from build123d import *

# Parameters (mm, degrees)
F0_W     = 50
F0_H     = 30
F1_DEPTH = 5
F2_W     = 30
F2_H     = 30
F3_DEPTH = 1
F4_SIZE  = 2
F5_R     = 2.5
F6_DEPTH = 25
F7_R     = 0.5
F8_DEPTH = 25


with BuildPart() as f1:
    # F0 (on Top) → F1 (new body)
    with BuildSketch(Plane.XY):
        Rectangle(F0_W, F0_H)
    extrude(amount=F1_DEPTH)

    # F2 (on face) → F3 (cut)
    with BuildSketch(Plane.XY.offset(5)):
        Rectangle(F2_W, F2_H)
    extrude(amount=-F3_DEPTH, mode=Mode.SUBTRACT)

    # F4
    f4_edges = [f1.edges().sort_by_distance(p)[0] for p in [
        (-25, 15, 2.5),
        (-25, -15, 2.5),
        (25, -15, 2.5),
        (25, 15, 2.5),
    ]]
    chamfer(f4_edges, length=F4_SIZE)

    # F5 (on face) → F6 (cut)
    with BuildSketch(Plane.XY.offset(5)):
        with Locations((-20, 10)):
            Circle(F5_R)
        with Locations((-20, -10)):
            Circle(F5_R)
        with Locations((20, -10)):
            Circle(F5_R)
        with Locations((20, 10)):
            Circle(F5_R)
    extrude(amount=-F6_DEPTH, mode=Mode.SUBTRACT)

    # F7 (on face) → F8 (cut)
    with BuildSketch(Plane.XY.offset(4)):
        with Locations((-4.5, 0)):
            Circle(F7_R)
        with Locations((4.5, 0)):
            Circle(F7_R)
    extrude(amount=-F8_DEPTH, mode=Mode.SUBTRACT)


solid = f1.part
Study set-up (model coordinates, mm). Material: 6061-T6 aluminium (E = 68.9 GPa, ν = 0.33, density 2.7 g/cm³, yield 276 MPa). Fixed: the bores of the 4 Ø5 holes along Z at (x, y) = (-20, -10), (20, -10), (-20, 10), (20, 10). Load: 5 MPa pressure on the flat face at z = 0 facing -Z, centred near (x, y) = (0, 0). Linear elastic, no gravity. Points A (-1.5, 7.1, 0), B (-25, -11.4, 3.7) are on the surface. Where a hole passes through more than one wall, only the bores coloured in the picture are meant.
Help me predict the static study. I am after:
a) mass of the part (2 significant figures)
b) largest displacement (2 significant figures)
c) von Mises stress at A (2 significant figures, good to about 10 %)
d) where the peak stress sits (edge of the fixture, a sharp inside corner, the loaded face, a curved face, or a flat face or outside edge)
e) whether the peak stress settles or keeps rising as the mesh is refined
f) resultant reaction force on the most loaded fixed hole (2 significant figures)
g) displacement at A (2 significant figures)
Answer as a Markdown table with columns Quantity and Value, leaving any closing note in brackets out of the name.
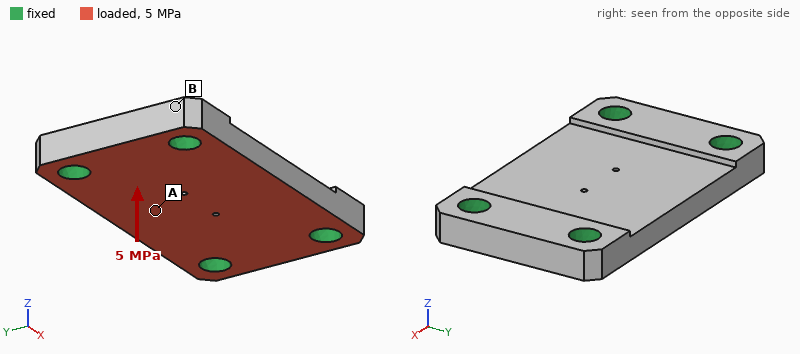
| Quantity | Value |
|---|---|
| mass of the part | 17 g |
| largest displacement | 68 µm |
| von Mises stress at A | 90 MPa |
| where the peak stress sits | edge of the fixture |
| whether the peak stress settles or keeps rising as the mesh is refined | keeps rising |
| resultant reaction force on the most loaded fixed hole | 1.8 kN |
| displacement at A | 64 µm |
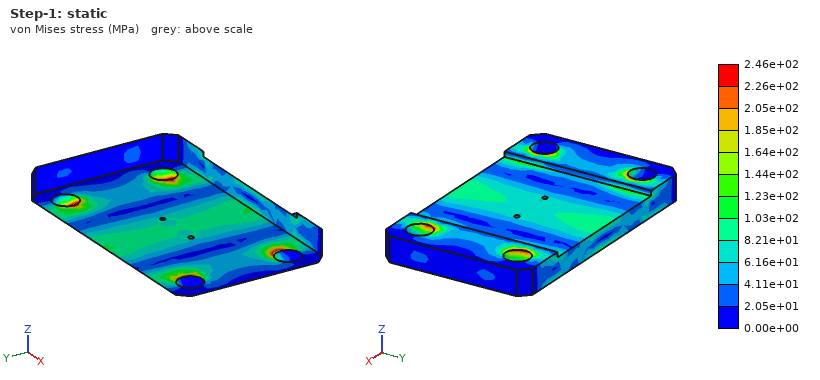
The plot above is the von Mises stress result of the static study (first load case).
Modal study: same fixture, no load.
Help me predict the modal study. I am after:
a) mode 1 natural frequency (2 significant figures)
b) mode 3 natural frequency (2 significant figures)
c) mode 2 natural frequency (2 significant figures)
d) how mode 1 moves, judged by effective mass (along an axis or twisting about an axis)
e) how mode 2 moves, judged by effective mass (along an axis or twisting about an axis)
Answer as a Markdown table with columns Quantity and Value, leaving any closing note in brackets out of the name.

| Quantity | Value |
|---|---|
| mode 1 natural frequency | 15 kHz |
| mode 3 natural frequency | 33 kHz |
| mode 2 natural frequency | 19 kHz |
| how mode 1 moves, judged by effective mass | along Z |
| how mode 2 moves, judged by effective mass | twisting about X |
